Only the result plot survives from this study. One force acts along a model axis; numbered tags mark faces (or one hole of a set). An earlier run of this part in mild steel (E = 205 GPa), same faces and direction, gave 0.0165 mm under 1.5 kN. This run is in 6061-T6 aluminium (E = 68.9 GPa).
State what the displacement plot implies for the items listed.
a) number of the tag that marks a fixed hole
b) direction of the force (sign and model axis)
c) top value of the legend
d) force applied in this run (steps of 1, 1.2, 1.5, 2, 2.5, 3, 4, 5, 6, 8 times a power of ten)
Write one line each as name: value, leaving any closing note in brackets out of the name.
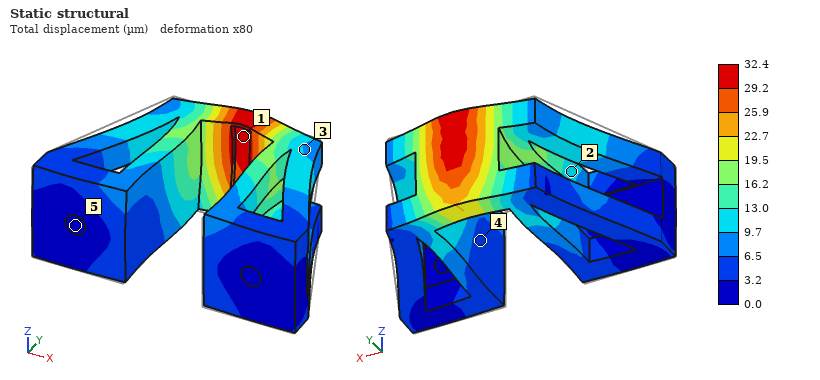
number of the tag that marks a fixed hole: 5
direction of the force: +Y
top value of the legend: 32.4 µm
force applied in this run: 1 kN
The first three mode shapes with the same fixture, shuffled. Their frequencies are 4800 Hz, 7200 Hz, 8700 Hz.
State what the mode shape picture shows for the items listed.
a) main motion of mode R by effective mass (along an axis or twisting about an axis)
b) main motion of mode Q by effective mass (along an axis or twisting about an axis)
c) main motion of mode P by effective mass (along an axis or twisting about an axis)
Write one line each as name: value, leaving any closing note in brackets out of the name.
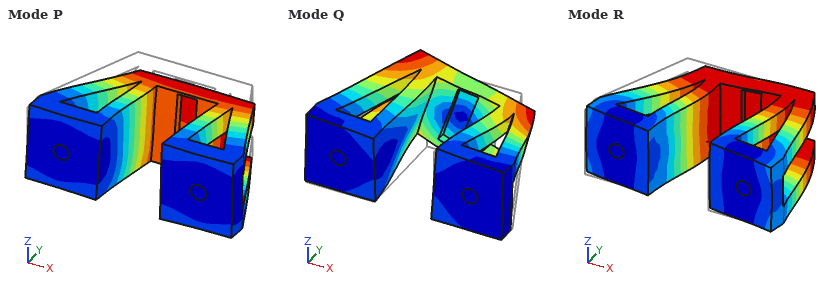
main motion of mode R by effective mass: along X
main motion of mode Q by effective mass: twisting about Y
main motion of mode P by effective mass: along Z
